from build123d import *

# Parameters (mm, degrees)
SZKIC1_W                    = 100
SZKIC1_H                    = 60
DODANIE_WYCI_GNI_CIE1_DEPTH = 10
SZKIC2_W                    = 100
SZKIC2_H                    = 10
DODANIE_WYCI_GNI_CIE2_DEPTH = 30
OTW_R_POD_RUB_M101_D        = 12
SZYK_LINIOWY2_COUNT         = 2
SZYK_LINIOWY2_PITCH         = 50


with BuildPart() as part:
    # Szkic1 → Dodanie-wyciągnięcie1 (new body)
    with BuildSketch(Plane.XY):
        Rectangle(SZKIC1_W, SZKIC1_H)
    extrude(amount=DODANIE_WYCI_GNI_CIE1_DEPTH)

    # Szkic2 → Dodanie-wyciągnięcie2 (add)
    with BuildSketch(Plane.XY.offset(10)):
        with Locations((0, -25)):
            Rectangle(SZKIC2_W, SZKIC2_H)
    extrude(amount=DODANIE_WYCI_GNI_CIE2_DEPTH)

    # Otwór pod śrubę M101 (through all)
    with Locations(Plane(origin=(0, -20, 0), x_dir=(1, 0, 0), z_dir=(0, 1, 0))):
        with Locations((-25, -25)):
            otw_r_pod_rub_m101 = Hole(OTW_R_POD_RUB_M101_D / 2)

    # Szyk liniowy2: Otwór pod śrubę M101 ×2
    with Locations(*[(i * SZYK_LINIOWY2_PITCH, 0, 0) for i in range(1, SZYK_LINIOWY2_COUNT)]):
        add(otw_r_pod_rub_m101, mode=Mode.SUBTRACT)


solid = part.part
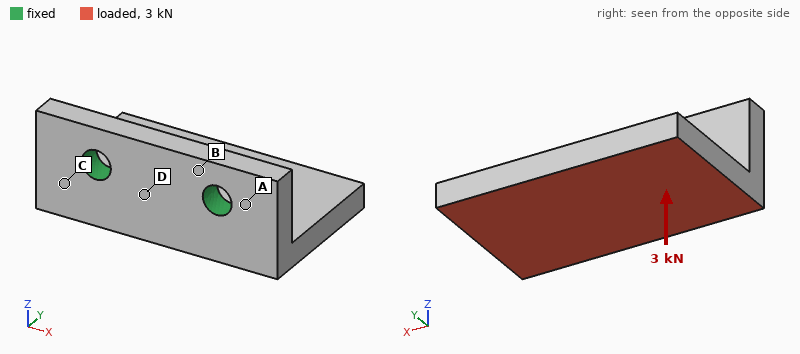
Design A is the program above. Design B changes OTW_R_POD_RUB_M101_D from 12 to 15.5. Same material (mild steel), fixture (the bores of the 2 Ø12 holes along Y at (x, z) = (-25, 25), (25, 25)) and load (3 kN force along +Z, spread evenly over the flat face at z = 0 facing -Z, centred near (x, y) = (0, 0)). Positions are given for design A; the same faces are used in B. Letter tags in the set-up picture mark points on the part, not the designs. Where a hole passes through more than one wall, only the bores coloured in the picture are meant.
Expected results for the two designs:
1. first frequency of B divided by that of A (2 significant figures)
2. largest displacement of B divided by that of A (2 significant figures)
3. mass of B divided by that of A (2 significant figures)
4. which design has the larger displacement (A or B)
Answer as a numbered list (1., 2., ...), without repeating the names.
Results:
1. 1.1
2. 0.91
3. 0.98
4. A
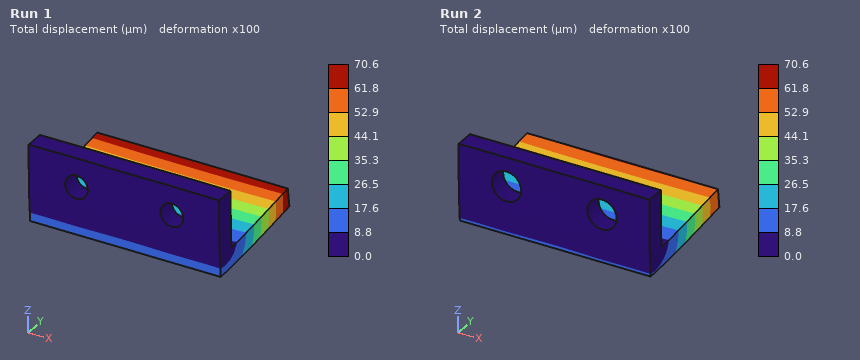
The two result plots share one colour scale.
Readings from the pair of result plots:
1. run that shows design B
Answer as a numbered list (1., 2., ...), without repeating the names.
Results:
1. Run 2
